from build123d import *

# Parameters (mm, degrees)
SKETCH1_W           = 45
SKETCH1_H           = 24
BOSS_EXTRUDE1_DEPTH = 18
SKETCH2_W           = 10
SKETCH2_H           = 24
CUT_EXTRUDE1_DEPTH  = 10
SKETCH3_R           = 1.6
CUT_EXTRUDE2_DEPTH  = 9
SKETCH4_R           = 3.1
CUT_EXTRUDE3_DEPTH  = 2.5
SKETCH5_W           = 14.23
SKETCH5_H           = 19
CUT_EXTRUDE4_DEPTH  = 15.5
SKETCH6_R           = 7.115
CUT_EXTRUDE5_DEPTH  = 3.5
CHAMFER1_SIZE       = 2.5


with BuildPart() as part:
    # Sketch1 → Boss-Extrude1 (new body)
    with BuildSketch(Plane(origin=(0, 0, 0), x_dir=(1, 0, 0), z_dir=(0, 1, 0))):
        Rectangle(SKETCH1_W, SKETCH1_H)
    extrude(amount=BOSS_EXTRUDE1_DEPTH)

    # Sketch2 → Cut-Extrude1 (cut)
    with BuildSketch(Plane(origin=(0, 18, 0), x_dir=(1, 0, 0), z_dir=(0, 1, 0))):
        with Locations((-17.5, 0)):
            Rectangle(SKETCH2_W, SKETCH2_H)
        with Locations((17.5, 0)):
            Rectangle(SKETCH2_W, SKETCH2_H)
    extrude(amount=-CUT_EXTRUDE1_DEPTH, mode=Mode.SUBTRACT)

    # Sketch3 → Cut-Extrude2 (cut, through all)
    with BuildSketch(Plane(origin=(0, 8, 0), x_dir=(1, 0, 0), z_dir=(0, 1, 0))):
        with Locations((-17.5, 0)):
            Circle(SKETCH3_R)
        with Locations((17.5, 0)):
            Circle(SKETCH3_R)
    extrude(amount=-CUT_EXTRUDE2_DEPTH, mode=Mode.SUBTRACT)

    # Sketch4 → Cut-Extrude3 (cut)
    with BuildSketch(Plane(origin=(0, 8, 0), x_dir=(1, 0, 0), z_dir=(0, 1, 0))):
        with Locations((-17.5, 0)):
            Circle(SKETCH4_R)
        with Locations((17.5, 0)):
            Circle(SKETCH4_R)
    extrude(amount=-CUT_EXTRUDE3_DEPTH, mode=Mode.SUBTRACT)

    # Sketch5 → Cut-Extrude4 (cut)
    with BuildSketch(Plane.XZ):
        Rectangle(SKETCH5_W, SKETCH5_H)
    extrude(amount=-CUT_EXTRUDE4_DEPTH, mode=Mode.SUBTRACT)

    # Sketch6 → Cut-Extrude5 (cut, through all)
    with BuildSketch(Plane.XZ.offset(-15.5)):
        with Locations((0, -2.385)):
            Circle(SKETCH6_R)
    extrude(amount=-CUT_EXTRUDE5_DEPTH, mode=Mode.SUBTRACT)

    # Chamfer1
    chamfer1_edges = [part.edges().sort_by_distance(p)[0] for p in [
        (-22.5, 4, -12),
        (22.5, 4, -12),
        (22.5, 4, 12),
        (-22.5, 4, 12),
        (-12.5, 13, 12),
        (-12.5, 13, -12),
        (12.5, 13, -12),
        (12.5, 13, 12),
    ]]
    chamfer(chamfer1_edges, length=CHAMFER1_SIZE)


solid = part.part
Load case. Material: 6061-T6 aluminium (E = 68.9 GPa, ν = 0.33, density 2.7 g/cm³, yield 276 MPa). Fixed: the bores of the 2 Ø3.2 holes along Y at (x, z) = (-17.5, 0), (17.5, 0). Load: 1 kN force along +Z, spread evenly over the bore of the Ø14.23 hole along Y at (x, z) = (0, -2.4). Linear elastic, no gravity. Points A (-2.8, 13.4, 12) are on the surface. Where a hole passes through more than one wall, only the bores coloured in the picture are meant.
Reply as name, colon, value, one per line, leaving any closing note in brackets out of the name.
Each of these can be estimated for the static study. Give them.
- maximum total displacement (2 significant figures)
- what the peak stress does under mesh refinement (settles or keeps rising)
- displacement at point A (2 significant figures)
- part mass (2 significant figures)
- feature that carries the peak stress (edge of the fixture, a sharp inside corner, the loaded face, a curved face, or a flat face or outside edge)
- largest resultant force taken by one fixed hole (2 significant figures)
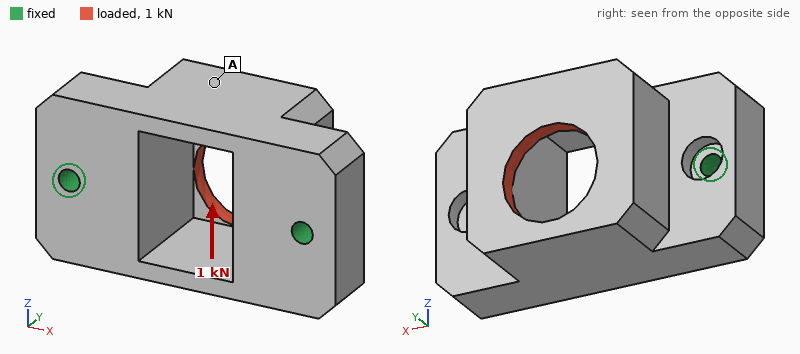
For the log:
maximum total displacement: 39 µm
what the peak stress does under mesh refinement: keeps rising
displacement at point A: 28 µm
part mass: 26 g
feature that carries the peak stress: edge of the fixture
largest resultant force taken by one fixed hole: 500 N
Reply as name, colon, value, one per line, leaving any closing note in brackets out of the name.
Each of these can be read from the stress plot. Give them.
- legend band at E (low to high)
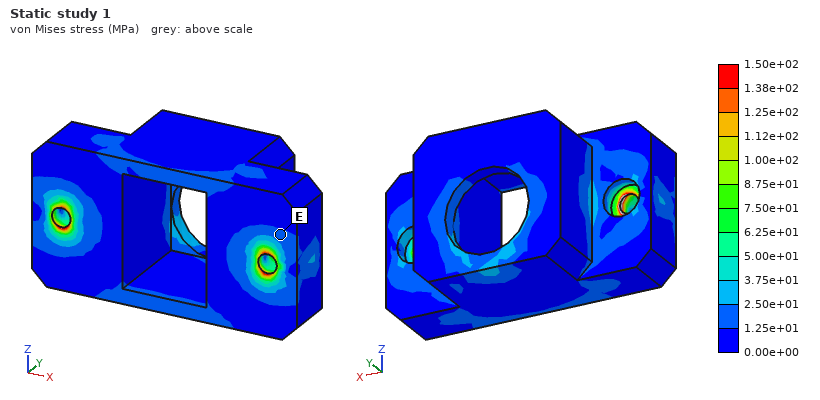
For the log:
legend band at E: 1.25e+01 to 2.50e+01 MPa
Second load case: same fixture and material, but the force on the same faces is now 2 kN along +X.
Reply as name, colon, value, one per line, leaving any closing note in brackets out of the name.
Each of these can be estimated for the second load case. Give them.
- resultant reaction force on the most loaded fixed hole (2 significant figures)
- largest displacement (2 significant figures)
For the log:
resultant reaction force on the most loaded fixed hole: 1.3 kN
largest displacement: 16 µm
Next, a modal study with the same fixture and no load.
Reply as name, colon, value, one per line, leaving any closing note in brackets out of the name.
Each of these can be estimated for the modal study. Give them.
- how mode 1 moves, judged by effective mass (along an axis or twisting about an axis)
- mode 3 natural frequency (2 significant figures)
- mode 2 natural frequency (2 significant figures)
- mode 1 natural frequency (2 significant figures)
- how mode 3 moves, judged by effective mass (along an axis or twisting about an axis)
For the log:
how mode 1 moves, judged by effective mass: along Z
mode 3 natural frequency: 20 kHz
mode 2 natural frequency: 17 kHz
mode 1 natural frequency: 9300 Hz
how mode 3 moves, judged by effective mass: along Y
